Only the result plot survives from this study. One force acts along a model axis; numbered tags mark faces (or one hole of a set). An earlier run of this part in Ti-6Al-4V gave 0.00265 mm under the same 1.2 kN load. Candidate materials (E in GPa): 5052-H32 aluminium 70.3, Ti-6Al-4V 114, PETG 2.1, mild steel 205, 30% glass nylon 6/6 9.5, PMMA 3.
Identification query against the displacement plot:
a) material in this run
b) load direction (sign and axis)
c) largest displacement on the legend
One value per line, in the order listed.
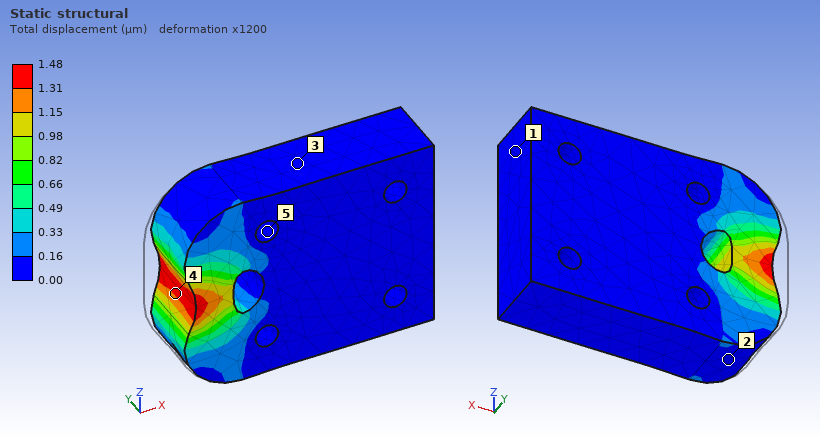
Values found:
mild steel
+X
1.48 µm
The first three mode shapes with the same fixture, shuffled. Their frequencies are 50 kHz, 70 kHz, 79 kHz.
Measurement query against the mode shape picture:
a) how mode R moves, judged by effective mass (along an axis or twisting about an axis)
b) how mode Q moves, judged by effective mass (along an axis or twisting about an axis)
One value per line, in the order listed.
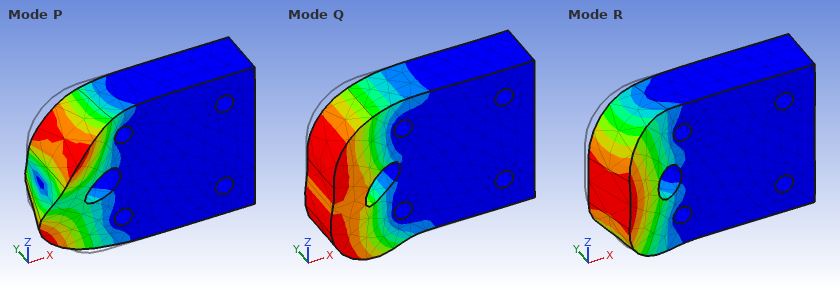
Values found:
along Y
along Z
